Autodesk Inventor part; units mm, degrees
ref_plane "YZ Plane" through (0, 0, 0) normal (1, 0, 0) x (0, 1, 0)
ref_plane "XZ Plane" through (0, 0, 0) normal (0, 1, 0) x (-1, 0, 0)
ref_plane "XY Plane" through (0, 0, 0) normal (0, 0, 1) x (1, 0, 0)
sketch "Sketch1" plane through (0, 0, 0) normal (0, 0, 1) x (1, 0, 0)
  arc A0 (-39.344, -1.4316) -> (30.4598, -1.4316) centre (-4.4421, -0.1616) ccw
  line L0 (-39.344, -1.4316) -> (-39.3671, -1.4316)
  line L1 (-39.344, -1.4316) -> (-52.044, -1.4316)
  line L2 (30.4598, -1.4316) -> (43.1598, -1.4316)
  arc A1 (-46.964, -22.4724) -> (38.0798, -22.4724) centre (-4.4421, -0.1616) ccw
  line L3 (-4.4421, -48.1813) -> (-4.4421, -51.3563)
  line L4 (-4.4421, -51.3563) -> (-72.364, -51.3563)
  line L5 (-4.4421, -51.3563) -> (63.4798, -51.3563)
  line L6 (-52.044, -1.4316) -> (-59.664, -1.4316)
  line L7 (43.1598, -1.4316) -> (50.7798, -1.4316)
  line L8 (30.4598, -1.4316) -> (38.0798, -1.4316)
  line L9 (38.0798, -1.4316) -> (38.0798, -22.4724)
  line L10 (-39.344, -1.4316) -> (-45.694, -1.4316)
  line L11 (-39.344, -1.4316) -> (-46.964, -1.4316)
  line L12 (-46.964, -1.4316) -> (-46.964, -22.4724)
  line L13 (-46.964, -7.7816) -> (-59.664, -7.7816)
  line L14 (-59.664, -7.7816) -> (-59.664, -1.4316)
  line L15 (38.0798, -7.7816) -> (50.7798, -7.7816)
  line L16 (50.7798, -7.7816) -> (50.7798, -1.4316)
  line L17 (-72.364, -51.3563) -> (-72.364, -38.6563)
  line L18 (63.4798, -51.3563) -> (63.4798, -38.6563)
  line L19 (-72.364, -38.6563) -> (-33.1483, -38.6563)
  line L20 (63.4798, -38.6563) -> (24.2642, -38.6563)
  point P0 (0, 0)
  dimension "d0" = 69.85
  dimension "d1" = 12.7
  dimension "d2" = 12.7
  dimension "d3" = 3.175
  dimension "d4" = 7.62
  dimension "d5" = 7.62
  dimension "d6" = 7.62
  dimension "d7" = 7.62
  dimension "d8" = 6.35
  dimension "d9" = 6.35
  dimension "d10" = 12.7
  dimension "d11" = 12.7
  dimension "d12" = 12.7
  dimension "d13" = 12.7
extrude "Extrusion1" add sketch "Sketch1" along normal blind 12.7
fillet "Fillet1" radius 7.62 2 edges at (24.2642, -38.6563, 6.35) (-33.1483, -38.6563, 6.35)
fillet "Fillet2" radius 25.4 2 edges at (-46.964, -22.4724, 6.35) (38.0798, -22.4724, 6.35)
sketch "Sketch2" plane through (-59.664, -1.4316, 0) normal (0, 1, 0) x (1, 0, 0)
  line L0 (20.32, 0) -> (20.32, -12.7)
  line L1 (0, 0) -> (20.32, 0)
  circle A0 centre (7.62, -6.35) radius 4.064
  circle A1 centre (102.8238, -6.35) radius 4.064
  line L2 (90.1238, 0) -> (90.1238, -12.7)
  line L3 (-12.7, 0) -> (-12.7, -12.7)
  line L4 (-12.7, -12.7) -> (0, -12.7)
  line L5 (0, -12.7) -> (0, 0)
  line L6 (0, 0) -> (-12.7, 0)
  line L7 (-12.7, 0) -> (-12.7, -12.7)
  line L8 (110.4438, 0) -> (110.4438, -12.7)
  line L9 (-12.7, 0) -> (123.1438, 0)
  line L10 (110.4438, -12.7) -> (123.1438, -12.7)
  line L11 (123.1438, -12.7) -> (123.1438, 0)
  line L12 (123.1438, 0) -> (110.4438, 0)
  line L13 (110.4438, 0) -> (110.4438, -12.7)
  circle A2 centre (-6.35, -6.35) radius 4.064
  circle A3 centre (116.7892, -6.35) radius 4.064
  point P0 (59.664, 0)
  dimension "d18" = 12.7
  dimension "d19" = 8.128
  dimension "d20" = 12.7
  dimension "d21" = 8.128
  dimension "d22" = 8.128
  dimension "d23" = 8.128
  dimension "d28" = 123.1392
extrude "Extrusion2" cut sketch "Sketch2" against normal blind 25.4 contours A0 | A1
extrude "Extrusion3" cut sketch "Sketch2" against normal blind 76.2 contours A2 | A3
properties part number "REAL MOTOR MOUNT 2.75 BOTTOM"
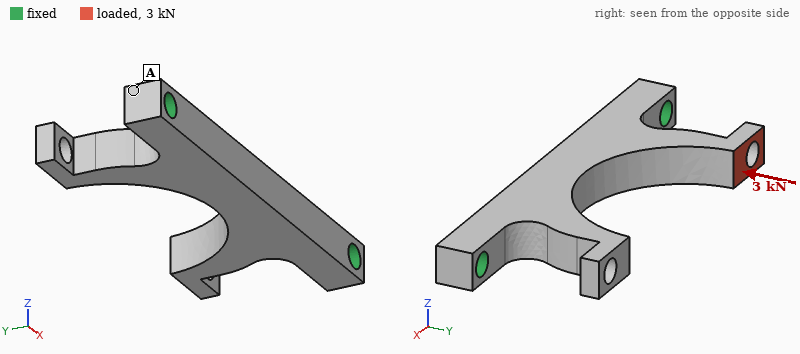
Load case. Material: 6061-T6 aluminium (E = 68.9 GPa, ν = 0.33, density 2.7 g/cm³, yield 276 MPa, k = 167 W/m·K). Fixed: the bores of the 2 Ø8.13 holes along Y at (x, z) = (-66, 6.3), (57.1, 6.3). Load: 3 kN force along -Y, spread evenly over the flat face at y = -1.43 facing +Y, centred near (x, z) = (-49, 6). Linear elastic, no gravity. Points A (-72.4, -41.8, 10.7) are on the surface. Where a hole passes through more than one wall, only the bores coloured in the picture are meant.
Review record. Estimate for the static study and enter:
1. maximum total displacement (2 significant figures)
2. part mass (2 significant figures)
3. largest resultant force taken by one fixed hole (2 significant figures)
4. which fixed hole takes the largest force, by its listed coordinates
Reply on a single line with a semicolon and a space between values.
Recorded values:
0.32 mm; 100 g; 2.9 kN; (-66, 6.3)
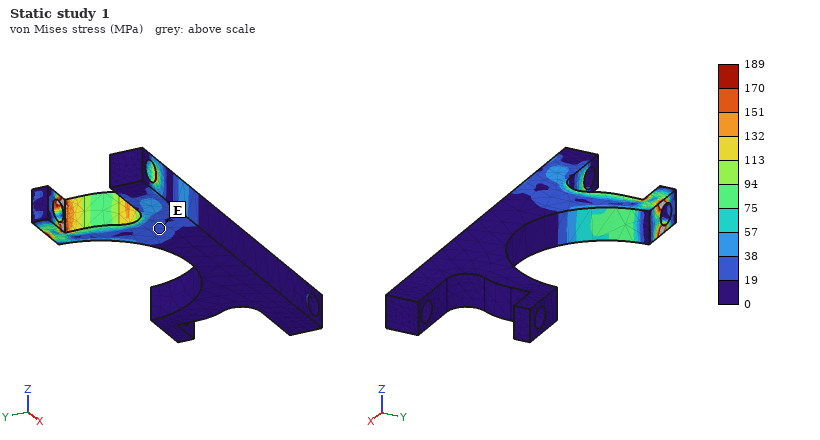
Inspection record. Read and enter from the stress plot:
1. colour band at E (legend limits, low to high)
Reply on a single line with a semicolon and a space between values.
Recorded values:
19 to 38 MPa
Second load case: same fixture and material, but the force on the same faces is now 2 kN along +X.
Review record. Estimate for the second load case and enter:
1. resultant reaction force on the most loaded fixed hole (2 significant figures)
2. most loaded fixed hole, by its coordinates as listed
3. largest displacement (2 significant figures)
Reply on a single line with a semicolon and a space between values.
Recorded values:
1.8 kN; (57.1, 6.3); 0.35 mm
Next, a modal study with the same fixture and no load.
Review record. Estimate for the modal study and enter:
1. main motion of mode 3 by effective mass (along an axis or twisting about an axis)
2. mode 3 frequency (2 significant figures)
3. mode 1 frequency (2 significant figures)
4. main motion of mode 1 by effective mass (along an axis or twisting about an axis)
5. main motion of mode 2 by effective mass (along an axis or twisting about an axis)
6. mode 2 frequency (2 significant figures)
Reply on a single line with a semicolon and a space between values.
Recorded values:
along Y; 3800 Hz; 2400 Hz; along Z; twisting about Y; 3700 Hz
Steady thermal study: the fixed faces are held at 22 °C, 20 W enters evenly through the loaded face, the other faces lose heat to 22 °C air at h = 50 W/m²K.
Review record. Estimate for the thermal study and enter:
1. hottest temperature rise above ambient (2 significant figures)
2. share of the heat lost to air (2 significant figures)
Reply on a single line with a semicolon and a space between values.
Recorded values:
47 K; 25 %
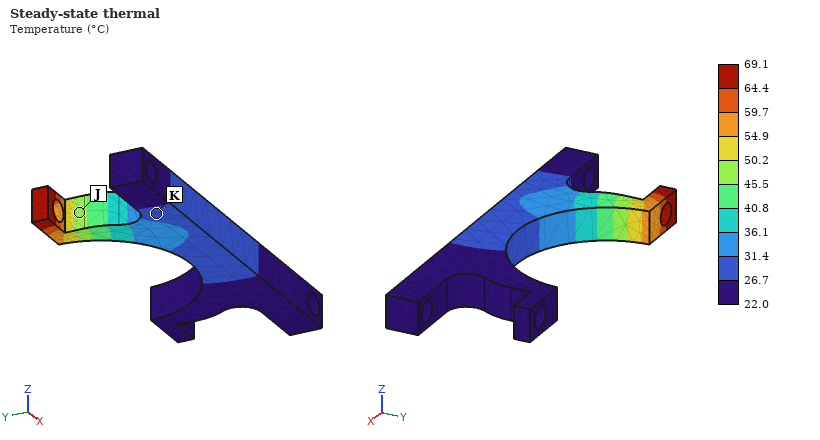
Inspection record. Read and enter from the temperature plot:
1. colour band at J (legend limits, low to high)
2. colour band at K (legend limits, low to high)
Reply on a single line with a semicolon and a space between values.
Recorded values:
45.5 to 50.2 °C; 26.7 to 31.4 °C
